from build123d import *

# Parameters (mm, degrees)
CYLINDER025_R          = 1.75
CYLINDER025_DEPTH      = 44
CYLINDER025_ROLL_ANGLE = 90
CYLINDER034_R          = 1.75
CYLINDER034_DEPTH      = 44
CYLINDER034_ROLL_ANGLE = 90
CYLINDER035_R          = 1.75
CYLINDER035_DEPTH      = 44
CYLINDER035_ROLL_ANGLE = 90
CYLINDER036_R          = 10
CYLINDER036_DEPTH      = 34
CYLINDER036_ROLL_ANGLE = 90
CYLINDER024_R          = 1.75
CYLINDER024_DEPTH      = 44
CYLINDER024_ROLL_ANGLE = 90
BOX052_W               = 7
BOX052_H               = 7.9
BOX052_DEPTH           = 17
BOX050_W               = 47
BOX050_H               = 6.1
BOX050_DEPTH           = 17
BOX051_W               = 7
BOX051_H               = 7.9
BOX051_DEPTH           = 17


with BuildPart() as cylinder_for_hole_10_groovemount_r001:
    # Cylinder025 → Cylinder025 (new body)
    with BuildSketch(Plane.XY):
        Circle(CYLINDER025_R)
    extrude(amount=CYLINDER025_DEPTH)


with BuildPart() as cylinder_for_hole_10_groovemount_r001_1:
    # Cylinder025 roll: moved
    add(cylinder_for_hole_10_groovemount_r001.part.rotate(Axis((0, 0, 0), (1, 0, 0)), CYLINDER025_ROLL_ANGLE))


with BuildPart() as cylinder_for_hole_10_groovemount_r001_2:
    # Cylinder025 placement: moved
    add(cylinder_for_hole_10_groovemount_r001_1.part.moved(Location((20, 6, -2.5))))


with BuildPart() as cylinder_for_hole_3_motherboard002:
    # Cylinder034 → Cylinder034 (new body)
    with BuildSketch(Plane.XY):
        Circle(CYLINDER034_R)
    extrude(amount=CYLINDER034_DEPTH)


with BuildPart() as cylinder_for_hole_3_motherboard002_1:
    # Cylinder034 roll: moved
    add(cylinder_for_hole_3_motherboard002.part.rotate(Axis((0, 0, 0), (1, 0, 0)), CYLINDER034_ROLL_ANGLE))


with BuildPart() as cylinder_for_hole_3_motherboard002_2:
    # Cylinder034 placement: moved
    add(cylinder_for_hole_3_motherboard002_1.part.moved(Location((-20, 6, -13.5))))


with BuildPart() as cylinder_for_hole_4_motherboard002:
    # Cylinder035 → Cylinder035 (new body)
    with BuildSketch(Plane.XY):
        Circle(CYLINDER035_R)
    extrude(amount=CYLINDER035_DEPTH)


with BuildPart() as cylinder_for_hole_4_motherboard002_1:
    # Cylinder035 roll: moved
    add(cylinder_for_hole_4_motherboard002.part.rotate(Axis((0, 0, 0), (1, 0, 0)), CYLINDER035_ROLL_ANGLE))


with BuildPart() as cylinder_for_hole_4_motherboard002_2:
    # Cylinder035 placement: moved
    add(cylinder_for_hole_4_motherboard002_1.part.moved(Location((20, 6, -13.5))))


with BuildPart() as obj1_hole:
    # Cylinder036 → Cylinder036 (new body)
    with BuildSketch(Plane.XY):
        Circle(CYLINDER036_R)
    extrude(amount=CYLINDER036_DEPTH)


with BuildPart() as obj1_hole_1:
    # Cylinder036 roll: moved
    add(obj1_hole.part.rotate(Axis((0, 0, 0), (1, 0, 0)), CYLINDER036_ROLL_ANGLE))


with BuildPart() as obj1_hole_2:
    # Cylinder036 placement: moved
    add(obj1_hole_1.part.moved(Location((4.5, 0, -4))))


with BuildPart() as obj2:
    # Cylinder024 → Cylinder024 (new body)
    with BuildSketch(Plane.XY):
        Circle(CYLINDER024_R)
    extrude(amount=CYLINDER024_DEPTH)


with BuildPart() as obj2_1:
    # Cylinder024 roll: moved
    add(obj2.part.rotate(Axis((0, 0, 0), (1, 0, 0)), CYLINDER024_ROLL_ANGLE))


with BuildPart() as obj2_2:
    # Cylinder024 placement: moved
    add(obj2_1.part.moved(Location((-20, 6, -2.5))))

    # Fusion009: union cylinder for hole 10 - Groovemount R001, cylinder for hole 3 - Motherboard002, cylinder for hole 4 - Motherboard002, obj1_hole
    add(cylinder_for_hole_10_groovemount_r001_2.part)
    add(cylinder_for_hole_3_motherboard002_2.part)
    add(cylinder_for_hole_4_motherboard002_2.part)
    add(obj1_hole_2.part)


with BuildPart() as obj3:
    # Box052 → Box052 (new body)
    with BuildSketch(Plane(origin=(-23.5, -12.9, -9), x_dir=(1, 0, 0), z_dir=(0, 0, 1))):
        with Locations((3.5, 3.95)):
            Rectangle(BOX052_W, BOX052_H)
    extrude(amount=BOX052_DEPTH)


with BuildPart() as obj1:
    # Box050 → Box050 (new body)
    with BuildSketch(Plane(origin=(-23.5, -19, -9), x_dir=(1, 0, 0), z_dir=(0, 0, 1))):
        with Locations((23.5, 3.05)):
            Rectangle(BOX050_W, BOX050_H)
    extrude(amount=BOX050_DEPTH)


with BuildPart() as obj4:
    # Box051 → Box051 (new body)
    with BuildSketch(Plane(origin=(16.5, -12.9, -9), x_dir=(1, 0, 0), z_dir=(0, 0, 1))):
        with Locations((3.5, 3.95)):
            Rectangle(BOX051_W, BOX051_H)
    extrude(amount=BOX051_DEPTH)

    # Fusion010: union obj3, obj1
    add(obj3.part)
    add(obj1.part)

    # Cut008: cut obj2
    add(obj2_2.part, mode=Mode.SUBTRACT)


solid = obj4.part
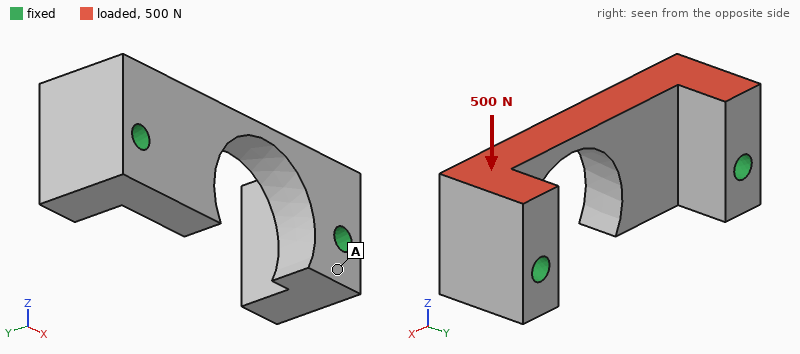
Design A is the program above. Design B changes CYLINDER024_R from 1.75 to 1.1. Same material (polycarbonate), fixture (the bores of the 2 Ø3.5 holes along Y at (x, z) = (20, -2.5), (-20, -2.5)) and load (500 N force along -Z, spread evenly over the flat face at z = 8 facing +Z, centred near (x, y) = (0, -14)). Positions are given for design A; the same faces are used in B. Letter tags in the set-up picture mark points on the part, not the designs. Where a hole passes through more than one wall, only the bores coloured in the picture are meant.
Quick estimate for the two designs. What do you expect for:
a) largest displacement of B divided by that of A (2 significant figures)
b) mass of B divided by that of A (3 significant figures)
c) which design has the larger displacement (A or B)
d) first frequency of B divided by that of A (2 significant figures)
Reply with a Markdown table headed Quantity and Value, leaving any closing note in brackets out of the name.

| Quantity | Value |
|---|---|
| largest displacement of B divided by that of A | 1.2 |
| mass of B divided by that of A | 1.02 |
| which design has the larger displacement | B |
| first frequency of B divided by that of A | 0.86 |
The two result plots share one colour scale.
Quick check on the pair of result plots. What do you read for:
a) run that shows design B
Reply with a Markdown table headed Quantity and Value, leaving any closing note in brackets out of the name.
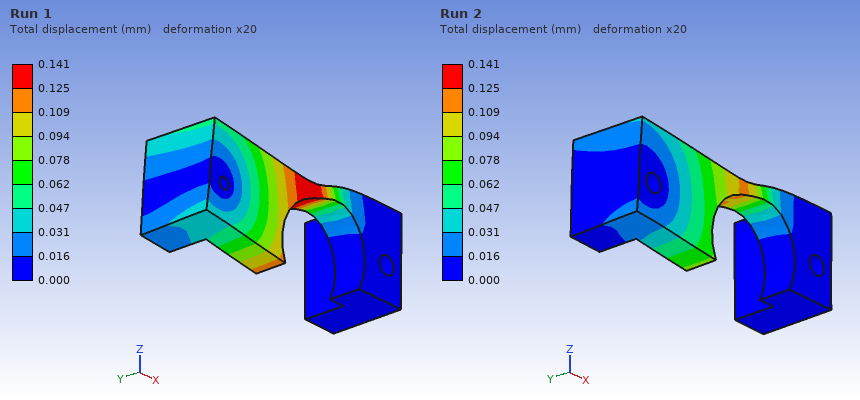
| Quantity | Value |
|---|---|
| run that shows design B | Run 1 |
